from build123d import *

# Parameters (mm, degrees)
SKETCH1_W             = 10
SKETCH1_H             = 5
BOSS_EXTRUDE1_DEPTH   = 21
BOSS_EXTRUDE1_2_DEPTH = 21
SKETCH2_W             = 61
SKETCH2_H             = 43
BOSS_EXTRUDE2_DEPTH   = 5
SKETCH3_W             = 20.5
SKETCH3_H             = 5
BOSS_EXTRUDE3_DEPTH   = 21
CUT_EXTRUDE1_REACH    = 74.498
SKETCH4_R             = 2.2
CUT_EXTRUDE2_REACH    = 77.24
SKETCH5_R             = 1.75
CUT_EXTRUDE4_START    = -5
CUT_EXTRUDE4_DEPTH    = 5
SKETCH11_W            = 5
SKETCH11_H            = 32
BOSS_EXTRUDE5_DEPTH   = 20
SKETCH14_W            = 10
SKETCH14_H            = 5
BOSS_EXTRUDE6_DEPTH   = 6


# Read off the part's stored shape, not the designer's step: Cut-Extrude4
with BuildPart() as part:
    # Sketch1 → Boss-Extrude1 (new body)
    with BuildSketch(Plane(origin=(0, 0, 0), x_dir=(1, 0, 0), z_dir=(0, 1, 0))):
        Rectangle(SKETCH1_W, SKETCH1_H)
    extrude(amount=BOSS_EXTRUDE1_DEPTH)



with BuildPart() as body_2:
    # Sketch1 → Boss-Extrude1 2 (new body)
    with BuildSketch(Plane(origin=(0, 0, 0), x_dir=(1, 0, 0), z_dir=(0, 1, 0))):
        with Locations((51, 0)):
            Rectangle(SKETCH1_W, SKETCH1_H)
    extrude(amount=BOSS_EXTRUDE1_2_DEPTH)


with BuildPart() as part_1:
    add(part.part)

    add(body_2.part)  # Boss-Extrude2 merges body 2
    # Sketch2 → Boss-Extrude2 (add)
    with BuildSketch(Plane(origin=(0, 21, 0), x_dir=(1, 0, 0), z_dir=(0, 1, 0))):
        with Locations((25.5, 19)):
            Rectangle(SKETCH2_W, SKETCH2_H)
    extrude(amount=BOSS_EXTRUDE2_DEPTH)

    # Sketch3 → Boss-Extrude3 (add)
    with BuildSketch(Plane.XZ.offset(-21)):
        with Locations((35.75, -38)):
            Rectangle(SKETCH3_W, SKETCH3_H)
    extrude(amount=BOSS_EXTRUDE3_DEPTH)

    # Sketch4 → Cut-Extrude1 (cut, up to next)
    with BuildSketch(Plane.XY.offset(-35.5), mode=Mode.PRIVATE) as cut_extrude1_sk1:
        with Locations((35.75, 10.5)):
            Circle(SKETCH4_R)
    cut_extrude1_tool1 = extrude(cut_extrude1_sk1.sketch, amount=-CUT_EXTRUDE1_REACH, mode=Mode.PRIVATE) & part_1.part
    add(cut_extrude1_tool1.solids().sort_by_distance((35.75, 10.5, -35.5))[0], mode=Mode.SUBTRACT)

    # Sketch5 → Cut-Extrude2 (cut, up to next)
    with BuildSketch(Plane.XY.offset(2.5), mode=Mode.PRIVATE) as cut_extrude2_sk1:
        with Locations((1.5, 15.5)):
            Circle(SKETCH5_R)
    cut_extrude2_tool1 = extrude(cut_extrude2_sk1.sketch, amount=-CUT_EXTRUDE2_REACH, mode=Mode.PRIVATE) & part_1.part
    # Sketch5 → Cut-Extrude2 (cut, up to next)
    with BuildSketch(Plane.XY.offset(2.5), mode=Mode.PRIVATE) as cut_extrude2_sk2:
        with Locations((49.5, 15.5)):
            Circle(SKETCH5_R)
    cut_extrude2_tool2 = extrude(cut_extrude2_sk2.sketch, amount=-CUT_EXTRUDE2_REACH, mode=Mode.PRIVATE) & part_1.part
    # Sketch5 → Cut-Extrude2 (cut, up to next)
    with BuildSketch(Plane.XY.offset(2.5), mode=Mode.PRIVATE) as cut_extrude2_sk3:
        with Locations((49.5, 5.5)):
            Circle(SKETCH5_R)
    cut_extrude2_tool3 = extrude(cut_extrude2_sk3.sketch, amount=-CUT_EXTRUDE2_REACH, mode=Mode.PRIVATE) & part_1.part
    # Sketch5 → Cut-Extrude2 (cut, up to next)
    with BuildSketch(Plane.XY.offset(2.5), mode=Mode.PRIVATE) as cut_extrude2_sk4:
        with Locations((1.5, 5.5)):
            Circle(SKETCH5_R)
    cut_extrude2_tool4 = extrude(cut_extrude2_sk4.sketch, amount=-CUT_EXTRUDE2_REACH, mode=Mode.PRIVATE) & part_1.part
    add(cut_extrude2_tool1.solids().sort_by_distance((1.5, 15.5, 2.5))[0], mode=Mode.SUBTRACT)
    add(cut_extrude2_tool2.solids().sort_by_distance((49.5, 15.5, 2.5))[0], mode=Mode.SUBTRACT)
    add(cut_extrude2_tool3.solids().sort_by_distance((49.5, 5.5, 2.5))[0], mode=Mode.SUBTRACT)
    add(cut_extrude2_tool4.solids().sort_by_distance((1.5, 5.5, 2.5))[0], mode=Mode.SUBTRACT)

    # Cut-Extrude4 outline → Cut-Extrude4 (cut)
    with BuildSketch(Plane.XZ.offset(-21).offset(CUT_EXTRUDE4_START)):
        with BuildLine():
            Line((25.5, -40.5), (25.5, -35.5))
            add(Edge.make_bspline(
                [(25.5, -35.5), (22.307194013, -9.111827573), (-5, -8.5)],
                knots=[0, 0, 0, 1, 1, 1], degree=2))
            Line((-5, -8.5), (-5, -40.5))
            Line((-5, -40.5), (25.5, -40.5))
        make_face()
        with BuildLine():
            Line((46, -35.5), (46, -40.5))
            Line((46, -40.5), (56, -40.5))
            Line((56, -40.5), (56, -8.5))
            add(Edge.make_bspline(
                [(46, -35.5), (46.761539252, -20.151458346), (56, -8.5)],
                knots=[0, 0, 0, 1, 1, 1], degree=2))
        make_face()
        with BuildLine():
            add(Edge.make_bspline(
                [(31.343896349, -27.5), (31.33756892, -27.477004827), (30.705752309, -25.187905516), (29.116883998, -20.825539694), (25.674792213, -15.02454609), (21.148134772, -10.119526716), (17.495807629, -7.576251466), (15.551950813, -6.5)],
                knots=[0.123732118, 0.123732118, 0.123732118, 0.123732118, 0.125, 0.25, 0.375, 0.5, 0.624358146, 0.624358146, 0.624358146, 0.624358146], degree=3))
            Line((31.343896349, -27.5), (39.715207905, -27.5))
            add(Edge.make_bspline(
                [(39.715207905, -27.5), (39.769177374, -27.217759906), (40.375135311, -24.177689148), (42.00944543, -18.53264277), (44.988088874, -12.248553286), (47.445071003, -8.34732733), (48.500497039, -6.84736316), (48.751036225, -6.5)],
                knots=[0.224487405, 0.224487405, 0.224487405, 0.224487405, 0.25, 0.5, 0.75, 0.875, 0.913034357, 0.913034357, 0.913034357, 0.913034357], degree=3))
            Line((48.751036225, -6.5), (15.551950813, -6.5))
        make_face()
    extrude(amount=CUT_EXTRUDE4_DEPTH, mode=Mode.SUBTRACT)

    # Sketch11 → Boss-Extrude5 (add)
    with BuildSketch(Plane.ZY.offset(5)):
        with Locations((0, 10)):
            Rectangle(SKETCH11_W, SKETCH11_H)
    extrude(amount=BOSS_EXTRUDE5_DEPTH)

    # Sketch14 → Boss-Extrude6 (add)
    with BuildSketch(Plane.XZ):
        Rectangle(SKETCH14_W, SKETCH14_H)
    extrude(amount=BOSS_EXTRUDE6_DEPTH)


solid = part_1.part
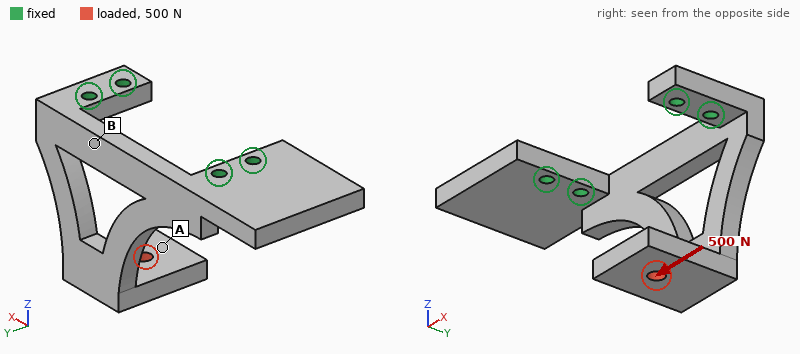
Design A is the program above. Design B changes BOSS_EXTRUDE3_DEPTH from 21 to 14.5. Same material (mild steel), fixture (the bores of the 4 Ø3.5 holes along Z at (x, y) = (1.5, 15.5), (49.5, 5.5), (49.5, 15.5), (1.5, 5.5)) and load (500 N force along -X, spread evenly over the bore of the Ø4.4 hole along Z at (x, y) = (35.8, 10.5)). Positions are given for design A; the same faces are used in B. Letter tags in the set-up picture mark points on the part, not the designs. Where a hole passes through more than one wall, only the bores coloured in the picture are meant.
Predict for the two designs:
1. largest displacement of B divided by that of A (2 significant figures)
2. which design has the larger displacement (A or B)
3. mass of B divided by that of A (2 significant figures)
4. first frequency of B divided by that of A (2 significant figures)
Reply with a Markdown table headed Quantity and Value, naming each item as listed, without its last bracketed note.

| Quantity | Value |
|---|---|
| largest displacement of B divided by that of A | 0.80 |
| which design has the larger displacement | A |
| mass of B divided by that of A | 0.95 |
| first frequency of B divided by that of A | 1.2 |
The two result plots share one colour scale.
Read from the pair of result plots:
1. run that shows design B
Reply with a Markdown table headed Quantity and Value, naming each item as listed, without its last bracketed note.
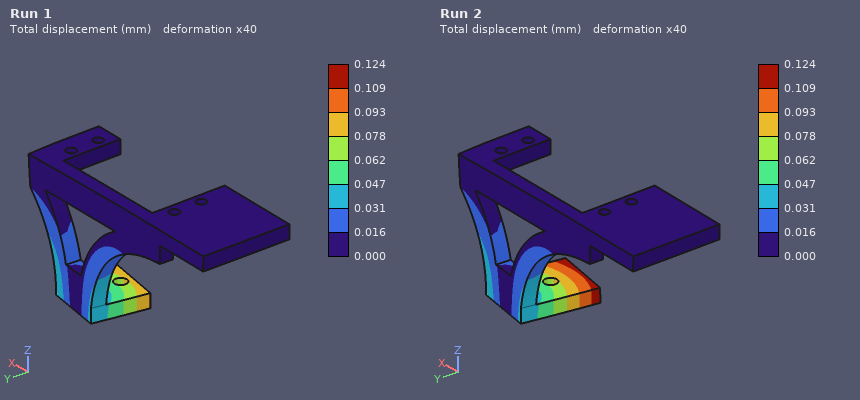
| Quantity | Value |
|---|---|
| run that shows design B | Run 1 |
